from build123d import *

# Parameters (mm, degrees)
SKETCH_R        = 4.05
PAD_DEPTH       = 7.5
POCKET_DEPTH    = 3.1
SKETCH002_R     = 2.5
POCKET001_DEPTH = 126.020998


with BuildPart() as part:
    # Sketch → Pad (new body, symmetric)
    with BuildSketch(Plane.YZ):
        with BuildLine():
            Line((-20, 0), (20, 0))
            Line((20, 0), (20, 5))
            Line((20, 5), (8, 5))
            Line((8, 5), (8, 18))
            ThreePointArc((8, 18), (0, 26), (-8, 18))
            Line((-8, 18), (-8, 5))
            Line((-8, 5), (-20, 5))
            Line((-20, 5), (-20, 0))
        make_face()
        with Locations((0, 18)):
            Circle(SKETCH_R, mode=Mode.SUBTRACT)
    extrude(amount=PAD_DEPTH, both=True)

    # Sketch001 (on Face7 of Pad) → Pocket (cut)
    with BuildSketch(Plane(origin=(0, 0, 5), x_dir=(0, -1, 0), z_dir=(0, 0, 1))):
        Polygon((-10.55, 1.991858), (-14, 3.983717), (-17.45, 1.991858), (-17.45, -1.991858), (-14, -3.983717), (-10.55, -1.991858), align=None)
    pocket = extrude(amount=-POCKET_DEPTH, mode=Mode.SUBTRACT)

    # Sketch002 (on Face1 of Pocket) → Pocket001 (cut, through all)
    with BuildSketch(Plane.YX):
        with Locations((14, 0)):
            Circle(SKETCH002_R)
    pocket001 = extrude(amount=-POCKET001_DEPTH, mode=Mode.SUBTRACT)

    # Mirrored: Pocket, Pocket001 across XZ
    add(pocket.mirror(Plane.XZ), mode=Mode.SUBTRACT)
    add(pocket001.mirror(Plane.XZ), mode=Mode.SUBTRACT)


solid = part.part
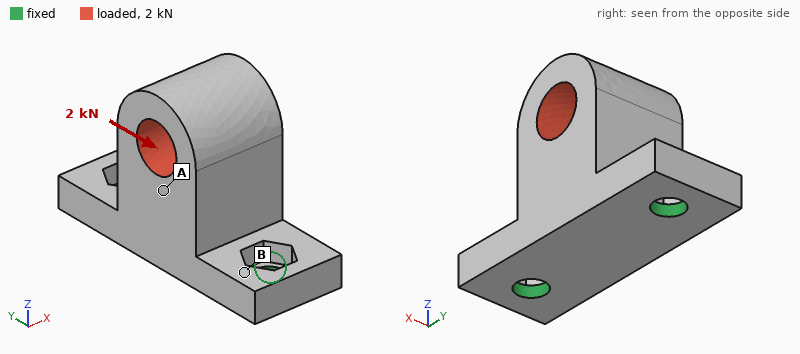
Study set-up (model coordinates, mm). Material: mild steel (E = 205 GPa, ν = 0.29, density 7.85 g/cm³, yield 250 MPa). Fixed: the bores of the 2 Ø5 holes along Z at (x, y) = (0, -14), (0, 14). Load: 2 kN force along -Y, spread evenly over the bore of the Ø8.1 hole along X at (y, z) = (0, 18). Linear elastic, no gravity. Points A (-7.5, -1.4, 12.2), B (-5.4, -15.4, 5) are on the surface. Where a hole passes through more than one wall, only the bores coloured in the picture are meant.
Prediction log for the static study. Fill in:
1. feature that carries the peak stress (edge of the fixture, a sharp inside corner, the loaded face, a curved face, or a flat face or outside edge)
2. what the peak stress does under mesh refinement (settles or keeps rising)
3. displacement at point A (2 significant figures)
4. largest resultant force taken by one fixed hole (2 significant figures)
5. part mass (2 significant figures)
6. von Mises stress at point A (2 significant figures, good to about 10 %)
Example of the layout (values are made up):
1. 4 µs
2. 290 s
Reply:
1. edge of the fixture
2. keeps rising
3. 6.3 µm
4. 1.7 kN
5. 51 g
6. 36 MPa
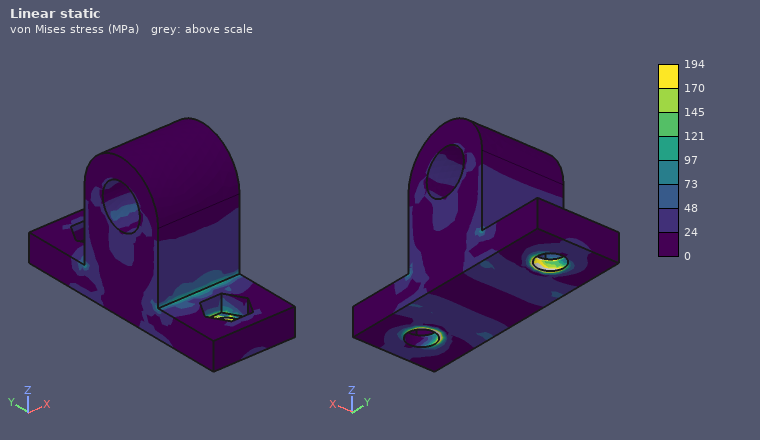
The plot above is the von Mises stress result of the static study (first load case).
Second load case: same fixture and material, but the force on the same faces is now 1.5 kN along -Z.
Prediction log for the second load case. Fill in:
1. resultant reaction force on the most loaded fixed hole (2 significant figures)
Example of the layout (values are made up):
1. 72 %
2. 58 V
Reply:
1. 940 N
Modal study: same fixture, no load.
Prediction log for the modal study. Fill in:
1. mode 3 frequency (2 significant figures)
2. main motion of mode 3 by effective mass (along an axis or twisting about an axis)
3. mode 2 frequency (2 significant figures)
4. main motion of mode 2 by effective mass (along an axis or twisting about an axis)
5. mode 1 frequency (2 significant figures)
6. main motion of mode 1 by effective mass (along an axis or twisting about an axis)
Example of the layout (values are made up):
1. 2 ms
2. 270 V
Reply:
1. 17 kHz
2. along Z
3. 13 kHz
4. along Y
5. 4700 Hz
6. along X
